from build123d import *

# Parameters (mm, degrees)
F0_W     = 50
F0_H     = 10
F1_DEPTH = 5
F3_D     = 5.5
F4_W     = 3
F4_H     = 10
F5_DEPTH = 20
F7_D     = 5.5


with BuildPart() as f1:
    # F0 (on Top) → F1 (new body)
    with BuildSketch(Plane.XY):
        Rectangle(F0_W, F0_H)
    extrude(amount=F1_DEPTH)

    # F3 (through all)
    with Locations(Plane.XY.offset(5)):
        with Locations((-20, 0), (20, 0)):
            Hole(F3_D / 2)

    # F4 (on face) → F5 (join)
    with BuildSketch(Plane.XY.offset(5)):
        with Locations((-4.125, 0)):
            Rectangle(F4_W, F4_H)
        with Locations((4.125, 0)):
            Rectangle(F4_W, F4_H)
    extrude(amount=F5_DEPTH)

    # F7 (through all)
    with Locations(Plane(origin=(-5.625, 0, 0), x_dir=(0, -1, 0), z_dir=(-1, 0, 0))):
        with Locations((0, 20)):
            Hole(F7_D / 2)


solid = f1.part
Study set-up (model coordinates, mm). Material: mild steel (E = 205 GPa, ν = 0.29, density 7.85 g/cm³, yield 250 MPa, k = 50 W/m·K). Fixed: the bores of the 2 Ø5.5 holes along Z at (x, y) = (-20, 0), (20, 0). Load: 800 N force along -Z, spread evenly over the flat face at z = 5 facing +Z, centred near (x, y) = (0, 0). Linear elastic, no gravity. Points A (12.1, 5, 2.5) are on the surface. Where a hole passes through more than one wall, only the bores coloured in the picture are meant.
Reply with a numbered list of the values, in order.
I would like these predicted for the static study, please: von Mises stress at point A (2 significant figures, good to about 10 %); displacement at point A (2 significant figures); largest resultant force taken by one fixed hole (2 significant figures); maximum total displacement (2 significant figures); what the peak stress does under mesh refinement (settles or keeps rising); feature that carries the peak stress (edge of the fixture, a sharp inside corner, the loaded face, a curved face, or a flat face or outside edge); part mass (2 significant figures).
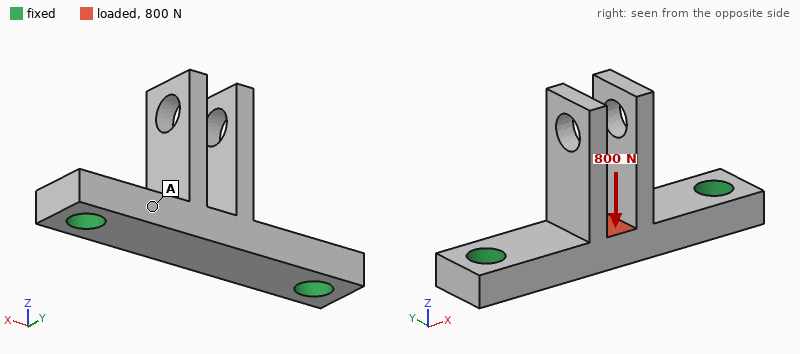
1. 24 MPa
2. 2.9 µm
3. 400 N
4. 17 µm
5. keeps rising
6. edge of the fixture
7. 26 g
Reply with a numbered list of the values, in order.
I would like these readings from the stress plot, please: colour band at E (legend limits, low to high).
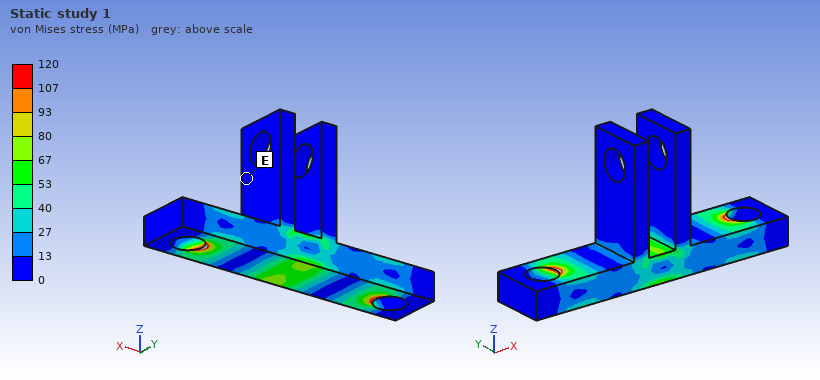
1. 0 to 13 MPa
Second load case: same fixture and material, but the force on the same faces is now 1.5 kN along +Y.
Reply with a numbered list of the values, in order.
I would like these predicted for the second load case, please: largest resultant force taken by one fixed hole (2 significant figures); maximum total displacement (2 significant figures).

1. 750 N
2. 32 µm
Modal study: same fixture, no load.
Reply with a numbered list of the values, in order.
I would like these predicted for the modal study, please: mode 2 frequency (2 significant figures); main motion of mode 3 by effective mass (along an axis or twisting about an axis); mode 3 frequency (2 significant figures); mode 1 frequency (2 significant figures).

1. 6000 Hz
2. along Y
3. 6800 Hz
4. 5800 Hz
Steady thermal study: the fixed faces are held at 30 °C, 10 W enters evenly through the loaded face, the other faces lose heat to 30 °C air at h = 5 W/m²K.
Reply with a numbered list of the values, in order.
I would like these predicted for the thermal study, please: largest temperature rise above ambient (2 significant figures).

1. 38 K
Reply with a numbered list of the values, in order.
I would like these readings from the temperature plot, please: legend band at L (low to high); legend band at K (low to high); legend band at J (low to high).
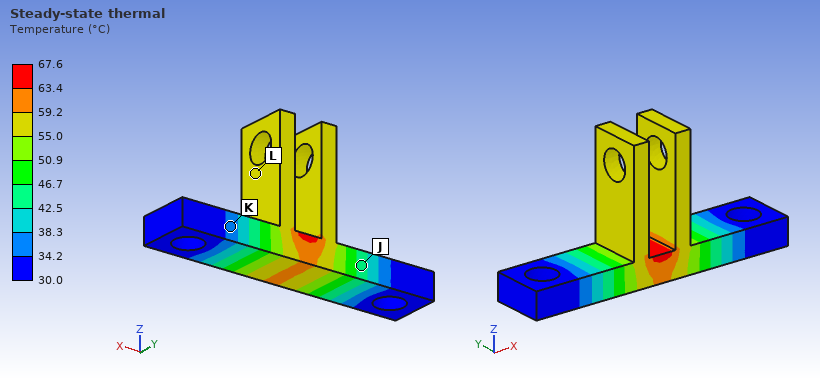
1. 55.0 to 59.2 °C
2. 34.2 to 38.3 °C
3. 42.5 to 46.7 °C
